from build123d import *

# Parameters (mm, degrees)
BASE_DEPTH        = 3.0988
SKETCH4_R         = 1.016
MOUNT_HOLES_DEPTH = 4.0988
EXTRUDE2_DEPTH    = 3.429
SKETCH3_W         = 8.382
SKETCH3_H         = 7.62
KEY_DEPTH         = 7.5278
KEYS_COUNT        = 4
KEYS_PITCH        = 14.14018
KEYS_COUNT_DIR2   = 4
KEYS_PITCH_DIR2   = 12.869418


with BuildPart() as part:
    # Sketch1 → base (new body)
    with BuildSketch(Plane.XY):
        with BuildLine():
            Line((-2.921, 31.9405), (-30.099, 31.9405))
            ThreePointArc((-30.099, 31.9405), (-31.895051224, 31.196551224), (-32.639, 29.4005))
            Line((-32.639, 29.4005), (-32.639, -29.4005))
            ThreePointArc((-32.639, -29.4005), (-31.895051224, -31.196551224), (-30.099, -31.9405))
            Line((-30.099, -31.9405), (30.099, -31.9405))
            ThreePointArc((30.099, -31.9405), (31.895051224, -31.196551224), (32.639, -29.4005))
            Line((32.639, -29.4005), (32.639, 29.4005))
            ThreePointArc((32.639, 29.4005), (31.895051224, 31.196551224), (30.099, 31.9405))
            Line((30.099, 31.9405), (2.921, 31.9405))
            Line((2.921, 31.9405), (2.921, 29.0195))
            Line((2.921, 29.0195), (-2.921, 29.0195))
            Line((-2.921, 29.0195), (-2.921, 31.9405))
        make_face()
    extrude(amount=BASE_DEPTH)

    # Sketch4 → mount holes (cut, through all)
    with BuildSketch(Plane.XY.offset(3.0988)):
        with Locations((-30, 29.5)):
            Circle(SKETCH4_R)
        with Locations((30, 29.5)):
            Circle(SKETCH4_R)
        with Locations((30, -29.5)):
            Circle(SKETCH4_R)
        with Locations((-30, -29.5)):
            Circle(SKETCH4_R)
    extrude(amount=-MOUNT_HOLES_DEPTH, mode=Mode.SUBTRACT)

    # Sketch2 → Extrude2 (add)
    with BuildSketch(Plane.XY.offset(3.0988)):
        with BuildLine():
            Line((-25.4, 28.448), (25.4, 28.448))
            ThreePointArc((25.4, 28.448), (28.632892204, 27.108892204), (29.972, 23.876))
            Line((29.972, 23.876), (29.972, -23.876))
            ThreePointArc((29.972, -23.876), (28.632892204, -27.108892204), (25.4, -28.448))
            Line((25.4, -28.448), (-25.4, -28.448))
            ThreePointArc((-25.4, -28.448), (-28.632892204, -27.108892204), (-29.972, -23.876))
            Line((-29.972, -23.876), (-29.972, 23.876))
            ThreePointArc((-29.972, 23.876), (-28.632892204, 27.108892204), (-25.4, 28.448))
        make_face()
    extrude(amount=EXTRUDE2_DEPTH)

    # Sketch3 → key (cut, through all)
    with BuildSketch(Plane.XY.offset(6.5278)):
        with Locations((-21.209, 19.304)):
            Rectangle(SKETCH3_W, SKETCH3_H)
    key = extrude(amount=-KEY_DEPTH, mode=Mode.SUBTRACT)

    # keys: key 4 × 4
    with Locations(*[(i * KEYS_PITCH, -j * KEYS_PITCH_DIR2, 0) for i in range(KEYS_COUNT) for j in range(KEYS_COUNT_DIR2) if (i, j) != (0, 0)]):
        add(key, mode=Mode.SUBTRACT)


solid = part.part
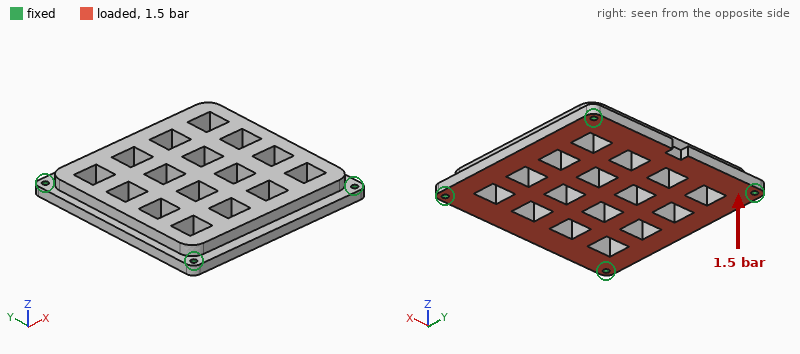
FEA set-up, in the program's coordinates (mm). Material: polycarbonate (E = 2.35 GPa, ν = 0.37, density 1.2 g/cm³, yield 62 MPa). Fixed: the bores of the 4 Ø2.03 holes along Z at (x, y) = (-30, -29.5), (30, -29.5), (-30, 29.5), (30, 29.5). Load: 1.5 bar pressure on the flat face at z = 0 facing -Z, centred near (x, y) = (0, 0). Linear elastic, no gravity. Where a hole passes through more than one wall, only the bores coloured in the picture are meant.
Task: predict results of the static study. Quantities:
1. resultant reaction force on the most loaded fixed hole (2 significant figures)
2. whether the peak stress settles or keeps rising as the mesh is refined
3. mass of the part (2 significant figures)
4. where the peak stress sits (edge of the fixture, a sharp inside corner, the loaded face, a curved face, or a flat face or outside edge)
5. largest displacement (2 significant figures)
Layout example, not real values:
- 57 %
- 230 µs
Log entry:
- 190 N
- keeps rising
- 21 g
- edge of the fixture
- 0.68 mm
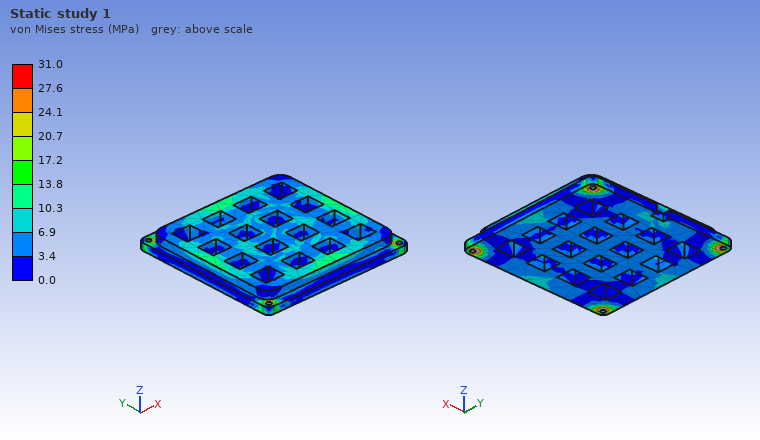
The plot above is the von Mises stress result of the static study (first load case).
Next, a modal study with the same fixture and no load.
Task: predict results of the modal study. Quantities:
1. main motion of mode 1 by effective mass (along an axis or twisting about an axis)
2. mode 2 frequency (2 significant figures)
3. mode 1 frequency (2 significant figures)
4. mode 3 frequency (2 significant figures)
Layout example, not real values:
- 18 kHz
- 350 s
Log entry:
- along Z
- 1800 Hz
- 1000 Hz
- 1800 Hz
